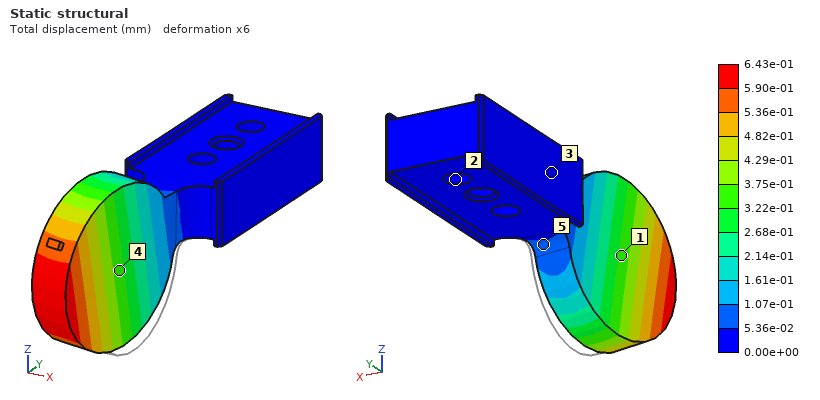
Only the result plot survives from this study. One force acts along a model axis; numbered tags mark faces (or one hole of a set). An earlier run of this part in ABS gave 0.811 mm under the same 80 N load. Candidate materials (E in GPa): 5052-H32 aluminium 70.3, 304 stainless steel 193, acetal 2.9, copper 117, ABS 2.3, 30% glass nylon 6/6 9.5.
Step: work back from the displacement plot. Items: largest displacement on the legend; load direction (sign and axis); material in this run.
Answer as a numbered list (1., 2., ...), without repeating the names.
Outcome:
1. 6.43e-01 mm
2. -X
3. acetal
